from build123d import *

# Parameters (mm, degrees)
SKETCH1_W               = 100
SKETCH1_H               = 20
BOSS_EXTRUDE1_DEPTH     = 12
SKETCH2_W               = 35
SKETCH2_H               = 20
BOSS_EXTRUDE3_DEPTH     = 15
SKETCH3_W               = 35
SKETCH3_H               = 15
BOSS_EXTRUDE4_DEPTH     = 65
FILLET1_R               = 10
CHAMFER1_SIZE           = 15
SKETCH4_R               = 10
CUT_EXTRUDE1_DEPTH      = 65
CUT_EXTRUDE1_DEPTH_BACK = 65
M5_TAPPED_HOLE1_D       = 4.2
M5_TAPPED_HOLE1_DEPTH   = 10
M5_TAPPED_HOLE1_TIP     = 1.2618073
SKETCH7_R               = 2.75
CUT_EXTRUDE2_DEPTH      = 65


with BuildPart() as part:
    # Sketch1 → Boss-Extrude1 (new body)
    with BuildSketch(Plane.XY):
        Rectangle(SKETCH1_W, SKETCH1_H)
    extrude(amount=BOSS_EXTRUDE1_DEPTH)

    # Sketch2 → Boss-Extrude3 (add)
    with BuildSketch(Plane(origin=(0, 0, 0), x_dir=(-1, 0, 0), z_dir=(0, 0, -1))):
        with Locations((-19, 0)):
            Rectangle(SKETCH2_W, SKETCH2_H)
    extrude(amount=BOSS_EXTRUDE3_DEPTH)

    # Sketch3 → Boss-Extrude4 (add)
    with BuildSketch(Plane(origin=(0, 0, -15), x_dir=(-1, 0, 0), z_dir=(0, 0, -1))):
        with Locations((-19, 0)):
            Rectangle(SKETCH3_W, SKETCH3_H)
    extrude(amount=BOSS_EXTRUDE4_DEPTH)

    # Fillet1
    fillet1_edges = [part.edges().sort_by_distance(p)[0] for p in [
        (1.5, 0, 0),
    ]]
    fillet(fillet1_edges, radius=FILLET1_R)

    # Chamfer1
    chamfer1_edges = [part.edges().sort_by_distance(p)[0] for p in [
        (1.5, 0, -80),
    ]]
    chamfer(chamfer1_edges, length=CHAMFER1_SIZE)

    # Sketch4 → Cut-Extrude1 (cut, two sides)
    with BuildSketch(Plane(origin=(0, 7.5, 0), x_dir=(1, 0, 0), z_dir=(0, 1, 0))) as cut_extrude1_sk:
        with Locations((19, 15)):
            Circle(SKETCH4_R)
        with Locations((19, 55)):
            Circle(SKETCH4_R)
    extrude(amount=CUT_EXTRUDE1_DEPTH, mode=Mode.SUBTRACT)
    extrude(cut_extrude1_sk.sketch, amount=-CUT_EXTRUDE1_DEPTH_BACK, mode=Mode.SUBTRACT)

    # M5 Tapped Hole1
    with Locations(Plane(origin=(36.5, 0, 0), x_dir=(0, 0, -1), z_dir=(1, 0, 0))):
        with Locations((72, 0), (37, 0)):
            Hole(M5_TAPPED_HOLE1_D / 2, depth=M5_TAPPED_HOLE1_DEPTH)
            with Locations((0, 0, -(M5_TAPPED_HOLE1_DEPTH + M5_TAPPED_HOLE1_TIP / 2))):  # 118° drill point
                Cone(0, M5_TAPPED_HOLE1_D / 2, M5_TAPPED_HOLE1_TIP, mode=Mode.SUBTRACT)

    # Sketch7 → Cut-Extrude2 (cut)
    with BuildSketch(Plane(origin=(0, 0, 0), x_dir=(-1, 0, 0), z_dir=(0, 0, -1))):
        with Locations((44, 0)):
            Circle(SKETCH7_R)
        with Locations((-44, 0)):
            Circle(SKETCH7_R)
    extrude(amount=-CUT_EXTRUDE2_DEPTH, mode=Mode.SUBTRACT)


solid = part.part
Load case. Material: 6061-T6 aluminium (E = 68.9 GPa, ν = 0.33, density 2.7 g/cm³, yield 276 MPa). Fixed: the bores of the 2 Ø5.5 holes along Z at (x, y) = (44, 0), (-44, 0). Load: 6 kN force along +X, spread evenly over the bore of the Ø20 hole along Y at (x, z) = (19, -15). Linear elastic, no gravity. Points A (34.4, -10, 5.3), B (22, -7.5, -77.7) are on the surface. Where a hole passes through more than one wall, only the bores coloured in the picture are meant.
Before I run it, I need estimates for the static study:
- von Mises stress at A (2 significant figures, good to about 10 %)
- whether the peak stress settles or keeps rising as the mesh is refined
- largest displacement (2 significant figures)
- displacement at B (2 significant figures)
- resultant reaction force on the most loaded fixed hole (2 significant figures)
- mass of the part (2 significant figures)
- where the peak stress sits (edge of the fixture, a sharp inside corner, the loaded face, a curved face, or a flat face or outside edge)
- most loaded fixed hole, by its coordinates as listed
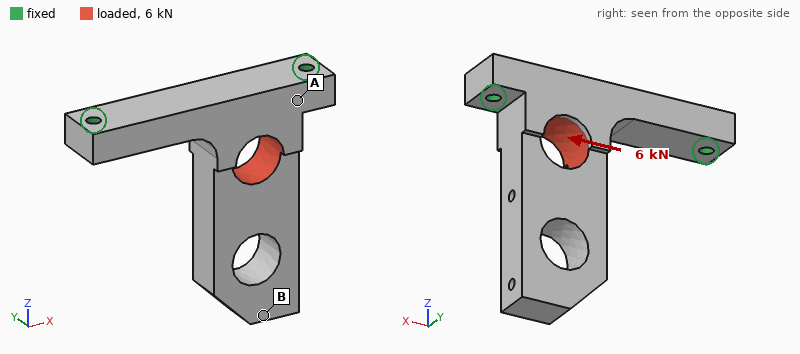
15 MPa
keeps rising
0.15 mm
0.15 mm
4.2 kN
150 g
edge of the fixture
(44, 0)
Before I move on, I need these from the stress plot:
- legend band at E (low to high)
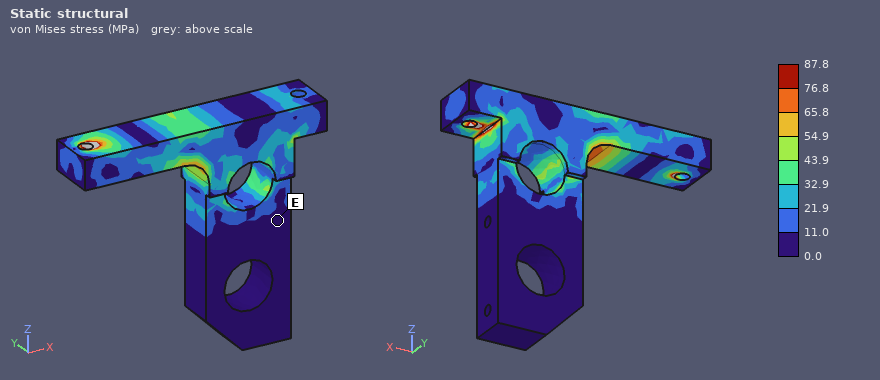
0.0 to 11.0 MPa
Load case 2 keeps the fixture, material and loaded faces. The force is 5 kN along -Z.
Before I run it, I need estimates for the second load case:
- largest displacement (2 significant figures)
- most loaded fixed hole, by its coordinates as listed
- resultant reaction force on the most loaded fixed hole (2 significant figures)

92 µm
(44, 0)
3.8 kN
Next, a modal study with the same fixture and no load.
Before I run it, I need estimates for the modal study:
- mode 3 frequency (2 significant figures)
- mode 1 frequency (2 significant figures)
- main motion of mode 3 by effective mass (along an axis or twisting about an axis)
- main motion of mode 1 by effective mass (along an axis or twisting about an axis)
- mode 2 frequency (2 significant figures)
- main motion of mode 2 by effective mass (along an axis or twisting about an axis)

5100 Hz
1200 Hz
along Y
along Y
2400 Hz
along X
